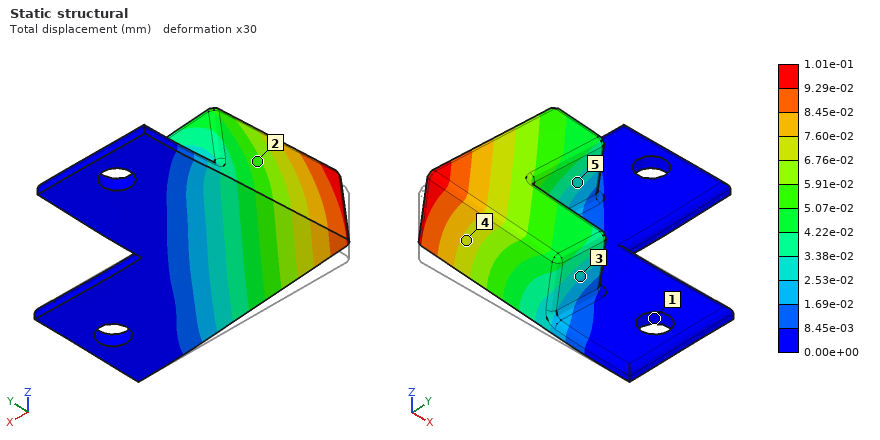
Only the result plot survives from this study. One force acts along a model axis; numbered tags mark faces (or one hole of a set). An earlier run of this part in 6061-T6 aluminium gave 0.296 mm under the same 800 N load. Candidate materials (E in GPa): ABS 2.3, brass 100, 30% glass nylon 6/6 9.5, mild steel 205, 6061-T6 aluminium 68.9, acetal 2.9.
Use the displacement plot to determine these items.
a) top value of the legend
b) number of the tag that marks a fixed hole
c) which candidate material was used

1.01e-01 mm
1
mild steel
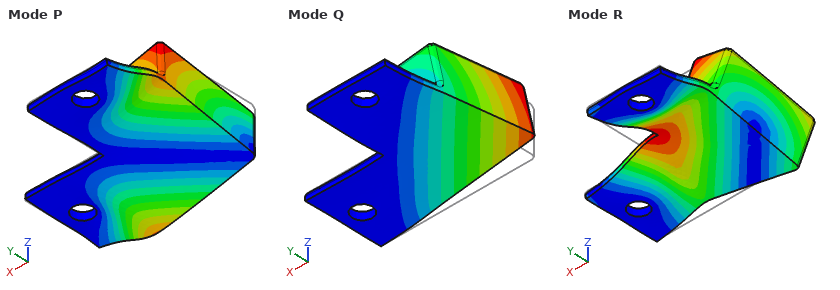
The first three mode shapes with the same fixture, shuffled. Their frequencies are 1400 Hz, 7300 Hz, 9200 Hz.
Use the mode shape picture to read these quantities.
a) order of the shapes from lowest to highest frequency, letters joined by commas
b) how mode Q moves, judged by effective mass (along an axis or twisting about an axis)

Q, P, R
along Z
